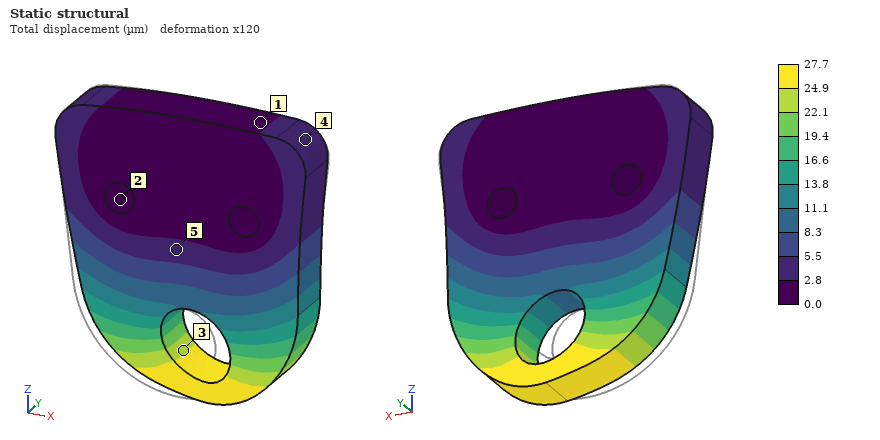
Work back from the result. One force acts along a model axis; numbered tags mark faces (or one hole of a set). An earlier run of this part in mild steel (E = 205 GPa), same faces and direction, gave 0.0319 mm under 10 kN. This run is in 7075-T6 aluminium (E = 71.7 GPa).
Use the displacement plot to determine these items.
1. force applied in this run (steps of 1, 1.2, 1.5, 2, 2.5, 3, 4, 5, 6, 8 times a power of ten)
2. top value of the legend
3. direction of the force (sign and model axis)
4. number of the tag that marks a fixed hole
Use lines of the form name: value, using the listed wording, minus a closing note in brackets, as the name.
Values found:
force applied in this run: 3 kN
top value of the legend: 27.7 µm
direction of the force: +X
number of the tag that marks a fixed hole: 2
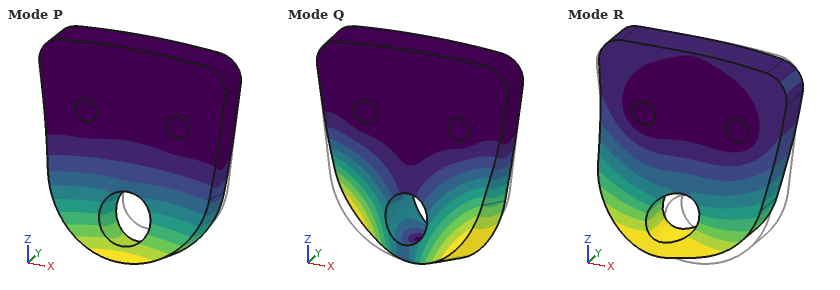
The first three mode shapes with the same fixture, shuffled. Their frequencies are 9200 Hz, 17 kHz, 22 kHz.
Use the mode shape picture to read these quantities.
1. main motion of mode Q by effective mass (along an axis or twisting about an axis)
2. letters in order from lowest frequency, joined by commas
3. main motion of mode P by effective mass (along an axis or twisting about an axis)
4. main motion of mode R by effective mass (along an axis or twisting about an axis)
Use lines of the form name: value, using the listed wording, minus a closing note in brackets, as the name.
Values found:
main motion of mode Q by effective mass: twisting about Z
letters in order from lowest frequency, joined by commas: P, Q, R
main motion of mode P by effective mass: along Y
main motion of mode R by effective mass: along X
